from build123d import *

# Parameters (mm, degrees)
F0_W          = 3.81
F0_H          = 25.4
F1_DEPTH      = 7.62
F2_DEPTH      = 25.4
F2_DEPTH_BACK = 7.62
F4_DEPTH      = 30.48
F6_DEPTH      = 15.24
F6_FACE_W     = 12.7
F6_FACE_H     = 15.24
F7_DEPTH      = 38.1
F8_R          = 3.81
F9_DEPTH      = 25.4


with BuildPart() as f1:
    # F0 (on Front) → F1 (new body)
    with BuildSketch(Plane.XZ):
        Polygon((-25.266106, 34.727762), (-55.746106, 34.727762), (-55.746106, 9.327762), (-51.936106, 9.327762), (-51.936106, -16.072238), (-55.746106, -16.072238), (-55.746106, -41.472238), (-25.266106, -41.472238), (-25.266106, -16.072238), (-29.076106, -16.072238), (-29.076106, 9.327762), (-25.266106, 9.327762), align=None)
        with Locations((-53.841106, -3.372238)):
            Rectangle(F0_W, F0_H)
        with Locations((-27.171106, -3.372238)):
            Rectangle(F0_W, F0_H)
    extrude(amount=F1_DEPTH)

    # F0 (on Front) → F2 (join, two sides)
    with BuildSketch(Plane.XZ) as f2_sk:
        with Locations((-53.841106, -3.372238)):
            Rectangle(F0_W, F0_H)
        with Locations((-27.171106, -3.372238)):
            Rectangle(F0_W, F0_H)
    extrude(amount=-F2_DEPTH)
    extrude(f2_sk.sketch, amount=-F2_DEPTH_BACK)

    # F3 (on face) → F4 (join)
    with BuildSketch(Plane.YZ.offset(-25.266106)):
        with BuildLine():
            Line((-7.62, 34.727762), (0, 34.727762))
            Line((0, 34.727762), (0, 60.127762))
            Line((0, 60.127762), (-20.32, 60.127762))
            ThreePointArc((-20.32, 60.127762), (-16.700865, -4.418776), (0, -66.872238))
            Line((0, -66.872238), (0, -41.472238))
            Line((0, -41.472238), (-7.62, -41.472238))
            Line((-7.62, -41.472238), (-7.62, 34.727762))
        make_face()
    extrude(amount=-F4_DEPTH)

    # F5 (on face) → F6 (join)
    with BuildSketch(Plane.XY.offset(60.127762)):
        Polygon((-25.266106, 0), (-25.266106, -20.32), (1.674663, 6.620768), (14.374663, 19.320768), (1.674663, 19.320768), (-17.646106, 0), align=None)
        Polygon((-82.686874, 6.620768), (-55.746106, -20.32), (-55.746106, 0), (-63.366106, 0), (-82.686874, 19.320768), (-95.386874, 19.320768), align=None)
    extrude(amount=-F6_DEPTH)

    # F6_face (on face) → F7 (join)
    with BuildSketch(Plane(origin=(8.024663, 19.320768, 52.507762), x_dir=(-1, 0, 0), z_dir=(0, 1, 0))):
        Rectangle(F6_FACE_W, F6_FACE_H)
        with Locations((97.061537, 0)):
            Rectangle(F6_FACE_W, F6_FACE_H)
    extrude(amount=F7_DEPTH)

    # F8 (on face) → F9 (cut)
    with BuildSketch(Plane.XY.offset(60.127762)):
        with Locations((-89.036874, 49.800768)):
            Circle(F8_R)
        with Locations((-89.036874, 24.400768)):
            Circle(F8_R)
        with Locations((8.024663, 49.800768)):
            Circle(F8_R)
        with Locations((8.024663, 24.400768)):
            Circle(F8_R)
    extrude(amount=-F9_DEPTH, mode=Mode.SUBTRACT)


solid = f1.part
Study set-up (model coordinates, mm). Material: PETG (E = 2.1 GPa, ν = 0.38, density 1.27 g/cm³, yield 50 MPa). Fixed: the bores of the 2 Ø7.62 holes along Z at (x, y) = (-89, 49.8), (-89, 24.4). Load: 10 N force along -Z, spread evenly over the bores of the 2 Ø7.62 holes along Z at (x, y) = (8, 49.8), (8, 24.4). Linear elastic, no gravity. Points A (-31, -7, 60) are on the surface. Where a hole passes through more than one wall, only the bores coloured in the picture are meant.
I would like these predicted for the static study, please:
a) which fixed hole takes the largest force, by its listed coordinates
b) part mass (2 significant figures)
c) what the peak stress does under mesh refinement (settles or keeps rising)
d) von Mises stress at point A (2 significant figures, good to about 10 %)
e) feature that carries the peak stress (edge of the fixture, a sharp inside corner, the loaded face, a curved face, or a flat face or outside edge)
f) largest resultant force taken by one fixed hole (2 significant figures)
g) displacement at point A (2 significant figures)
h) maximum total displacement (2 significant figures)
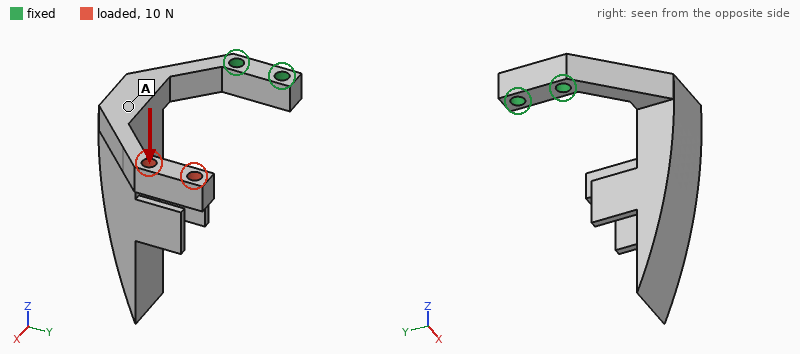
(-89, 24.4)
110 g
keeps rising
0.58 MPa
edge of the fixture
9.7 N
0.52 mm
2.1 mm
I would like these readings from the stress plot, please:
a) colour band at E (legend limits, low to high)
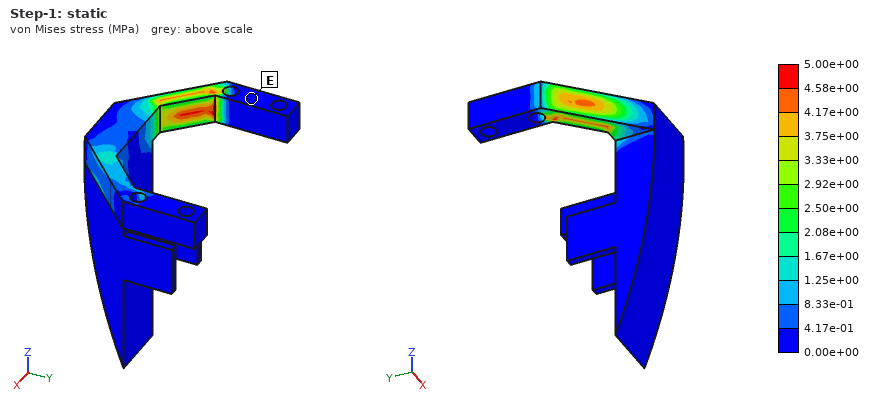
0.00e+00 to 4.17e-01 MPa
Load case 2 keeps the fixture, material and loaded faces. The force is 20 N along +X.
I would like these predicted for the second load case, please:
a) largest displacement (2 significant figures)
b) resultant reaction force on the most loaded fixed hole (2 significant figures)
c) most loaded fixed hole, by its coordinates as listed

1.9 mm
19 N
(-89, 24.4)
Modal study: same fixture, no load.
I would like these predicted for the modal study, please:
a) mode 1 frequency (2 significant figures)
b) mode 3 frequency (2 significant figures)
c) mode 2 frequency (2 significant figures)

56 Hz
120 Hz
79 Hz
